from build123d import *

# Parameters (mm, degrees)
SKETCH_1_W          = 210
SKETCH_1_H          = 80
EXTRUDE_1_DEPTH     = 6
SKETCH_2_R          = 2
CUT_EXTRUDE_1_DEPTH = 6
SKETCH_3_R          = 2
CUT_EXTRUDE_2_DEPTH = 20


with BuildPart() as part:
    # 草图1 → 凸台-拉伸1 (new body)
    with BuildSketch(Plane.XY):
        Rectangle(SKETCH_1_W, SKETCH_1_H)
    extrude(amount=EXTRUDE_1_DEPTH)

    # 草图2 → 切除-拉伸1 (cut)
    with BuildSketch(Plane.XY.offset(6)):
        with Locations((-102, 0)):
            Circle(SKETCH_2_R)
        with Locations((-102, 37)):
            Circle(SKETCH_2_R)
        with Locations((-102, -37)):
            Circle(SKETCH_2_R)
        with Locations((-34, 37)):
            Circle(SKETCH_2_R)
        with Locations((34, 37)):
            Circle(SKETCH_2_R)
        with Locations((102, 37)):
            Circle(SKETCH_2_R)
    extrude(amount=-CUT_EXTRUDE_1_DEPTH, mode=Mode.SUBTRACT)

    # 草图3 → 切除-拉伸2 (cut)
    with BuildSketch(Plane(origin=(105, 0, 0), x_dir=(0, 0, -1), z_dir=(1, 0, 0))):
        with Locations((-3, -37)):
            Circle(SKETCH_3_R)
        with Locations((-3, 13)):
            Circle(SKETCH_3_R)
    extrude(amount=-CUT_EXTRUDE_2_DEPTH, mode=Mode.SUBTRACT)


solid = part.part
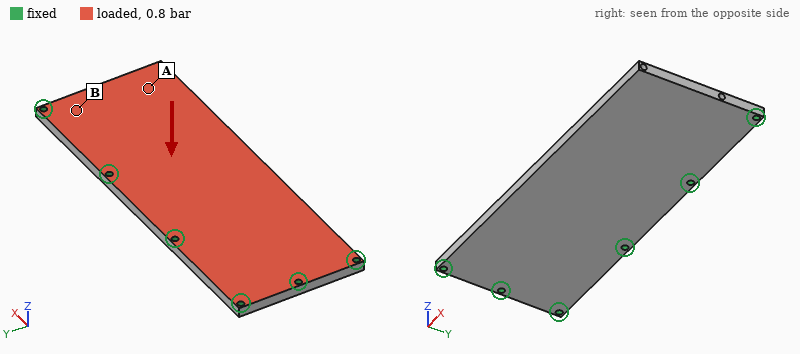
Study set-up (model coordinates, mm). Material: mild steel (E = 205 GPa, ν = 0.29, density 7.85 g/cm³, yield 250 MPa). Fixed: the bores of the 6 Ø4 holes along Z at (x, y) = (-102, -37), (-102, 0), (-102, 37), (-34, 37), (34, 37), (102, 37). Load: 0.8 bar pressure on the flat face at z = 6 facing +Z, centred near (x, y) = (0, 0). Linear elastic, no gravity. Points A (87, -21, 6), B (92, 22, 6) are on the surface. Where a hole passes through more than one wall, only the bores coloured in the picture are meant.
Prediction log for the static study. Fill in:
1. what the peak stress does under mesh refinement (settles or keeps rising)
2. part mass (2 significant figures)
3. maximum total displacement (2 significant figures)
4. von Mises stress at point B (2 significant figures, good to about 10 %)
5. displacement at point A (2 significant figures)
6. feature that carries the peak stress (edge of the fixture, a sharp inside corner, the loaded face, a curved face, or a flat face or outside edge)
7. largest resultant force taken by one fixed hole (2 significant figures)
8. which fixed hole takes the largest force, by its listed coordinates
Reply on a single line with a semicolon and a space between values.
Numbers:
keeps rising; 780 g; 0.15 mm; 26 MPa; 0.11 mm; edge of the fixture; 480 N; (34, 37)
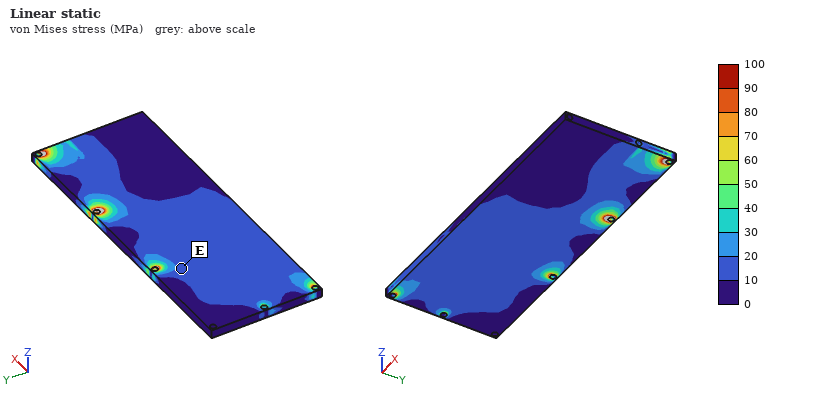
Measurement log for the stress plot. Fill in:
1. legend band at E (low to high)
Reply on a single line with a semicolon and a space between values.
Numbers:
10 to 20 MPa
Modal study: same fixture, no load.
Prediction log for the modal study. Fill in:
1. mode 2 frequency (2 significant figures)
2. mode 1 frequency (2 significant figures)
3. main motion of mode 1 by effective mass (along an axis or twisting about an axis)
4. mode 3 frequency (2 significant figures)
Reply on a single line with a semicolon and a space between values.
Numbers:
1400 Hz; 720 Hz; along Z; 2700 Hz
